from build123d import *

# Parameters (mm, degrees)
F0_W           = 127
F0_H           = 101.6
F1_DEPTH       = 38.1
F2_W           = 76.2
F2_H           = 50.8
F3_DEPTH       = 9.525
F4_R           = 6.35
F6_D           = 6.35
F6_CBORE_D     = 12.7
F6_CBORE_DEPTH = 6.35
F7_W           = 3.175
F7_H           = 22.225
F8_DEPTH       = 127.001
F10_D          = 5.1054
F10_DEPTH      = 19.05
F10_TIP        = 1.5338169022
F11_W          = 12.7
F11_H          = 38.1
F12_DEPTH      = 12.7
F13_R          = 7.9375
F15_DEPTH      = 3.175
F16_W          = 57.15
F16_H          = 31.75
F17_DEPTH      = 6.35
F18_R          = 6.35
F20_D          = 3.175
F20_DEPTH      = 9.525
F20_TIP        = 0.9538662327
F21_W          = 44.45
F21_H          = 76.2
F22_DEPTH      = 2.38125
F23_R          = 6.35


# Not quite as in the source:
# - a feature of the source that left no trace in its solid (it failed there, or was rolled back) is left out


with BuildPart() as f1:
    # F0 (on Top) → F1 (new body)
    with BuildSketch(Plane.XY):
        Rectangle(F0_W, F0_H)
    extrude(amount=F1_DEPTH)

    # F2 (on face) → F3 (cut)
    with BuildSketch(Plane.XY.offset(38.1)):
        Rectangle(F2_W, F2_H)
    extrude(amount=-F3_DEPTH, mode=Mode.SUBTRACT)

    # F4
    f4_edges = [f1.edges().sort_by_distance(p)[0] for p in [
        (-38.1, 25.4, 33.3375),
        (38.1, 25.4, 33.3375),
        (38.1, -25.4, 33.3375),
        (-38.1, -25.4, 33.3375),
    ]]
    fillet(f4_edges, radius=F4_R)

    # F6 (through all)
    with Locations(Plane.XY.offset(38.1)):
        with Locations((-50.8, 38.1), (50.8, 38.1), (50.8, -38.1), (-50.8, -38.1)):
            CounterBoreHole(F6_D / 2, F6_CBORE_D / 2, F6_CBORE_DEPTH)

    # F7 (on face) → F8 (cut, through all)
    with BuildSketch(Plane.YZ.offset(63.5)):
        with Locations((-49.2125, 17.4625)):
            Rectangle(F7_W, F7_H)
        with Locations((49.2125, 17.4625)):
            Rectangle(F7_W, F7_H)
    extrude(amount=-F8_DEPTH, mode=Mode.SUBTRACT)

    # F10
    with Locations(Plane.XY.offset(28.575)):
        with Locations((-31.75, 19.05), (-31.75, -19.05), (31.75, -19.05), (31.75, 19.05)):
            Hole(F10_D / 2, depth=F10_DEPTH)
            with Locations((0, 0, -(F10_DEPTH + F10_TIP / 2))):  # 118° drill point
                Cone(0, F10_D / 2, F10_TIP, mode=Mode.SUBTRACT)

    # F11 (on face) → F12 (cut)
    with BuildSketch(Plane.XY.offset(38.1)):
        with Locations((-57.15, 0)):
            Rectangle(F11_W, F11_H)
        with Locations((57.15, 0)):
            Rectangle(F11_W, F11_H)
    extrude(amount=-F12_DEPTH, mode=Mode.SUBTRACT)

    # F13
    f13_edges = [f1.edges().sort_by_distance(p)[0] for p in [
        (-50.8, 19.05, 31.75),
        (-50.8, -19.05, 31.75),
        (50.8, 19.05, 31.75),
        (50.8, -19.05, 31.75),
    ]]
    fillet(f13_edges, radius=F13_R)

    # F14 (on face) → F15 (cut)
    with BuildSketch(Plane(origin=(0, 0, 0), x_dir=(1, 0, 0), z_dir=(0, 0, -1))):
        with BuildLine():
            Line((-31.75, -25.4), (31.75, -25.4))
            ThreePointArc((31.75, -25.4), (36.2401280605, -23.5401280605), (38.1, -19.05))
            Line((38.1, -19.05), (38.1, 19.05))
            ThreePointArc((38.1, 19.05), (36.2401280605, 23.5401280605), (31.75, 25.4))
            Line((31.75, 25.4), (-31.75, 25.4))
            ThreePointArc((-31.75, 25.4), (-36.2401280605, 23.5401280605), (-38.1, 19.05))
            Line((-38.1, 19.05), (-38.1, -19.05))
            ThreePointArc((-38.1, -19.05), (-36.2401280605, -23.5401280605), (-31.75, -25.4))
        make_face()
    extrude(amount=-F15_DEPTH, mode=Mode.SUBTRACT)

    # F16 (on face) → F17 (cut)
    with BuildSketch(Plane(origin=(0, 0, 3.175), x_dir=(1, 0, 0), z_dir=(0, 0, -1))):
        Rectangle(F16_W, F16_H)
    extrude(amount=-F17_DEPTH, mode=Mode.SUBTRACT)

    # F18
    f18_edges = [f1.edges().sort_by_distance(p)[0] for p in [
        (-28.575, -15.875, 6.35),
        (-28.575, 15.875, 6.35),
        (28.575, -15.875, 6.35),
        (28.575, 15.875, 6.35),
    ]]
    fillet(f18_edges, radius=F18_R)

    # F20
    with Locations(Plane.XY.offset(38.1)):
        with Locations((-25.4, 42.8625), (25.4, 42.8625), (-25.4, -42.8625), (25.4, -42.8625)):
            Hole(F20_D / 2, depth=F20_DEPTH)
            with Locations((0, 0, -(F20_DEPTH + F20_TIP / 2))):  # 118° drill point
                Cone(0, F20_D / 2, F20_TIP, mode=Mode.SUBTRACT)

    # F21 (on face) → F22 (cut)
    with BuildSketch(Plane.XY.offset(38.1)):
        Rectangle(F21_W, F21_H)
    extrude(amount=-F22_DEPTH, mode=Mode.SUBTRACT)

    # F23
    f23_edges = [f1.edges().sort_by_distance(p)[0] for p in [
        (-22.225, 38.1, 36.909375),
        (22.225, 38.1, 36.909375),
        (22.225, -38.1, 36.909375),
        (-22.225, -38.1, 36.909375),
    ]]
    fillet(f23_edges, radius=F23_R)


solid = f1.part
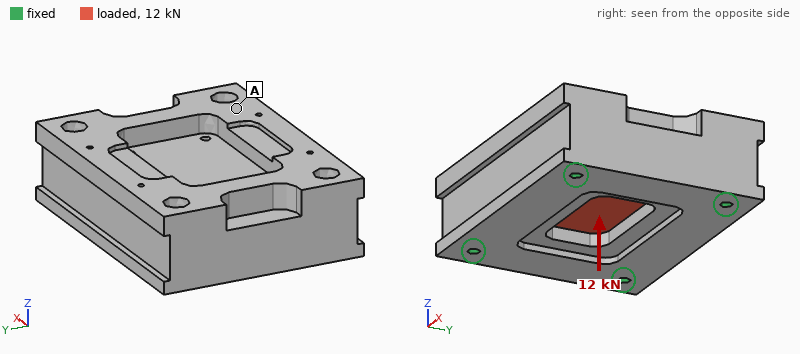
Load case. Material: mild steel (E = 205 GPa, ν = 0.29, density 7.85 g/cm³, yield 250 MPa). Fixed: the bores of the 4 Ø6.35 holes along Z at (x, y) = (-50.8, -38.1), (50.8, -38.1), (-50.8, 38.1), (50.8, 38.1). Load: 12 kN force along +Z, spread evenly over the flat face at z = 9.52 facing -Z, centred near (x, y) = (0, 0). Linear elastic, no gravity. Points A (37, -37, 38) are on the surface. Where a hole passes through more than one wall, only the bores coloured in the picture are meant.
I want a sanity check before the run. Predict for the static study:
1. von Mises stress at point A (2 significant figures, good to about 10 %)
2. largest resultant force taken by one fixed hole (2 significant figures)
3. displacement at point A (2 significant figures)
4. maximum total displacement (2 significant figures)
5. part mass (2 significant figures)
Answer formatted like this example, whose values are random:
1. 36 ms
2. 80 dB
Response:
1. 4.6 MPa
2. 3.0 kN
3. 1.5 µm
4. 5.7 µm
5. 3.1 kg
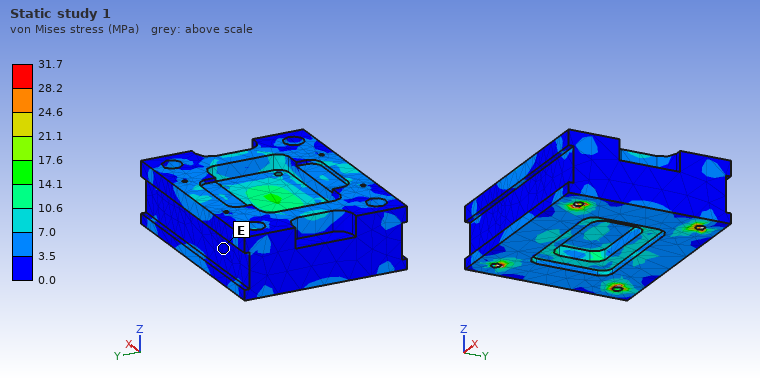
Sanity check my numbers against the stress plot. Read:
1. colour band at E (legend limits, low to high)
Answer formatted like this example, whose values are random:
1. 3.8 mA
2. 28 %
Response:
1. 0.0 to 3.5 MPa
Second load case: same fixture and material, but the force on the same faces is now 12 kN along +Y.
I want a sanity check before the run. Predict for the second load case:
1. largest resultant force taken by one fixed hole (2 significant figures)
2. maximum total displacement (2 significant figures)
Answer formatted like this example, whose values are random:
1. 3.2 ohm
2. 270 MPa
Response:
1. 3.5 kN
2. 2.4 µm
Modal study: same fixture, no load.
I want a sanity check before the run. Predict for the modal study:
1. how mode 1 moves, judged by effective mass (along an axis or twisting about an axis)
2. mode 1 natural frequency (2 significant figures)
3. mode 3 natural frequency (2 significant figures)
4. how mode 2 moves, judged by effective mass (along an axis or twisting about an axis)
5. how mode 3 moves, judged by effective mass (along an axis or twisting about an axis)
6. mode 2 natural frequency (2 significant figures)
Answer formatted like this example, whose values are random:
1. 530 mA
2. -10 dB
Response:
1. along Z
2. 8400 Hz
3. 12 kHz
4. twisting about X
5. along Y
6. 11 kHz
